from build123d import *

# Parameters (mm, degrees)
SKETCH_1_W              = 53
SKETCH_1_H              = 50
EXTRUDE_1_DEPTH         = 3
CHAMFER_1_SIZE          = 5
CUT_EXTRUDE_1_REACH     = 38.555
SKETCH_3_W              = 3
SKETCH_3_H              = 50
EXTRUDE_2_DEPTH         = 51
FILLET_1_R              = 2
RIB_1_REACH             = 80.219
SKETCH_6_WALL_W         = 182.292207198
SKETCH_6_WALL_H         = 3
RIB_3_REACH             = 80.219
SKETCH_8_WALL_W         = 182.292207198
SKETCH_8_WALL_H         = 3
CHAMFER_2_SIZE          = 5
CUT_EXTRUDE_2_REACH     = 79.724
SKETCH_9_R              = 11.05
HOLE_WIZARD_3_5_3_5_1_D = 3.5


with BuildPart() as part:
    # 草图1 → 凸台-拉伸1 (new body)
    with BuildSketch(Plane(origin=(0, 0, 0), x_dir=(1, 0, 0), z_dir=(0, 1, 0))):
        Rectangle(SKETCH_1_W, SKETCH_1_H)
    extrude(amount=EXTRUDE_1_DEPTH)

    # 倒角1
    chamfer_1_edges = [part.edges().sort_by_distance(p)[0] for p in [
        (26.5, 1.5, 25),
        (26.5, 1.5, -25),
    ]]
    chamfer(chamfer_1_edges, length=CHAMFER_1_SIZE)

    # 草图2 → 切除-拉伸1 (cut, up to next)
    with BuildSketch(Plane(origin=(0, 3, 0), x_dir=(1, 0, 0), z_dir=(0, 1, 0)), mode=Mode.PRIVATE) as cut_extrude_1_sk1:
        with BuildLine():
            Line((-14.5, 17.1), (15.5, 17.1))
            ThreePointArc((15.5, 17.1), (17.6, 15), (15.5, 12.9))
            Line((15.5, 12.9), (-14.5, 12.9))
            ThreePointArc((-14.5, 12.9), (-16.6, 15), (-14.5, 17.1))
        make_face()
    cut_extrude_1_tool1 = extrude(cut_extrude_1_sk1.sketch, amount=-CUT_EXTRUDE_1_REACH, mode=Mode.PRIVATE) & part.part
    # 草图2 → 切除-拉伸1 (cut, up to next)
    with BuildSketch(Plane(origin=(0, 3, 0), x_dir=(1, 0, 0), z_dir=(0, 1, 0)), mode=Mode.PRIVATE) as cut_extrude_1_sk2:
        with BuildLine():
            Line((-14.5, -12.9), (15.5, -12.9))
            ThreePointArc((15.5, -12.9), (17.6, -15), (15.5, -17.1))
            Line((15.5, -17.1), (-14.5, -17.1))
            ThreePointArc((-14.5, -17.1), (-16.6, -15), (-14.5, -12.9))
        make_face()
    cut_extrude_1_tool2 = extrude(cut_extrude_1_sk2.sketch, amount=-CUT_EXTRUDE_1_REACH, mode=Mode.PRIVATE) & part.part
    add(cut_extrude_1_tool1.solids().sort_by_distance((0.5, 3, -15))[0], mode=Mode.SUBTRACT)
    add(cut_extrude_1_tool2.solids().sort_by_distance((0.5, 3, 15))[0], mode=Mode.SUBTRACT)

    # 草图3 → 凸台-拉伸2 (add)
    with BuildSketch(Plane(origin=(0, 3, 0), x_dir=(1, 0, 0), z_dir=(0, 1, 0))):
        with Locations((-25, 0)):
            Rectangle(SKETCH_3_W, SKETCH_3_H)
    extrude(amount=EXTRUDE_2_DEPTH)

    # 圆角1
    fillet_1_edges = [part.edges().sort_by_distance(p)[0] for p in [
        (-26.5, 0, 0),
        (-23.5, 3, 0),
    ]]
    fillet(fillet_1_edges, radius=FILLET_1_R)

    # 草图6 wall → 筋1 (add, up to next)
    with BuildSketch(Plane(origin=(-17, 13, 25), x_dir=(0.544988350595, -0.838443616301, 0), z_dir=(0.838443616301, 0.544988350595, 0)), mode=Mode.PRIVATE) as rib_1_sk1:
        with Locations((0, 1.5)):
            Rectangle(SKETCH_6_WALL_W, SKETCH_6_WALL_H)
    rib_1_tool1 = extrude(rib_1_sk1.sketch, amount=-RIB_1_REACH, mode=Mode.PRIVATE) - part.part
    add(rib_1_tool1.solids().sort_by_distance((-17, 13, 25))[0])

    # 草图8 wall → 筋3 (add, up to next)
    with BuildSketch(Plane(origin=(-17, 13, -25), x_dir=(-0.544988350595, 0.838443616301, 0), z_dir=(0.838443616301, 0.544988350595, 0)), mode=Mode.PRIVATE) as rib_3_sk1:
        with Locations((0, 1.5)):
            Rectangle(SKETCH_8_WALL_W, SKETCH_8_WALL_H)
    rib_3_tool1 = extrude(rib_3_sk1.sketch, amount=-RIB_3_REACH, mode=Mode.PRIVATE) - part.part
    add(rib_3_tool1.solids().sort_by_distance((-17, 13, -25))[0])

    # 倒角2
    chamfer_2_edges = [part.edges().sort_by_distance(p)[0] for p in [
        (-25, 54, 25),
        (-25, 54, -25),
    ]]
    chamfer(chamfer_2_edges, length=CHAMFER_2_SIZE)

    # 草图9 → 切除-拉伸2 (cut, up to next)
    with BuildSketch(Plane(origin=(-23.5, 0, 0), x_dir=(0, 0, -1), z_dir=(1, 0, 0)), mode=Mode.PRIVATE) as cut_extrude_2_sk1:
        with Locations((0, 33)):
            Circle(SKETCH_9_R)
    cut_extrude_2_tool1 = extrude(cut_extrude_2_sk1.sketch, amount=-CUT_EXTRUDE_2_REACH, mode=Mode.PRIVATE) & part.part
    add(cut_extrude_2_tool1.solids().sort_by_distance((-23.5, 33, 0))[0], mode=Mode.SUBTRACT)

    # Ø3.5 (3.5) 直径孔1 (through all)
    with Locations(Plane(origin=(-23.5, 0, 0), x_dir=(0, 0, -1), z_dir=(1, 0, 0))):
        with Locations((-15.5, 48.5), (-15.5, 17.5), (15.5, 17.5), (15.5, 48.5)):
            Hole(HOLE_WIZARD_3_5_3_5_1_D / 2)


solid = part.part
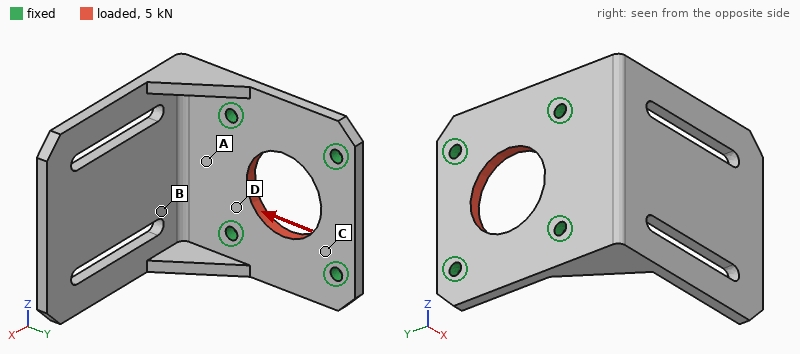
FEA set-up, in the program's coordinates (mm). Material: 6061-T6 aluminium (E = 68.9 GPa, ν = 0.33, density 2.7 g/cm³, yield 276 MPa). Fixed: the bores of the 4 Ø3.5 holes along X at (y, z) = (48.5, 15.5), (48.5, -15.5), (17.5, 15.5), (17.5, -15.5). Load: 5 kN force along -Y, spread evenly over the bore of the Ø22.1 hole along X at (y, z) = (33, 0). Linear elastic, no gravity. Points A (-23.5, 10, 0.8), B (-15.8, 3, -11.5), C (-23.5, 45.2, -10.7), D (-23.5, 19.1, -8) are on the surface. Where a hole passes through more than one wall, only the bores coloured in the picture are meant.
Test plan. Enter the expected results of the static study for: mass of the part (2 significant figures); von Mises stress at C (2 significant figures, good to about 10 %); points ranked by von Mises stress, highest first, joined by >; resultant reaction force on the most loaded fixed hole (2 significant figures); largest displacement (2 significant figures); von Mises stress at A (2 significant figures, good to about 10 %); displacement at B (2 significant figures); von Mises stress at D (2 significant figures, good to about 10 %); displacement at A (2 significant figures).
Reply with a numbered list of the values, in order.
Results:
1. 38 g
2. 36 MPa
3. C > D > A > B
4. 1.3 kN
5. 15 µm
6. 11 MPa
7. 3.7 µm
8. 21 MPa
9. 5.6 µm
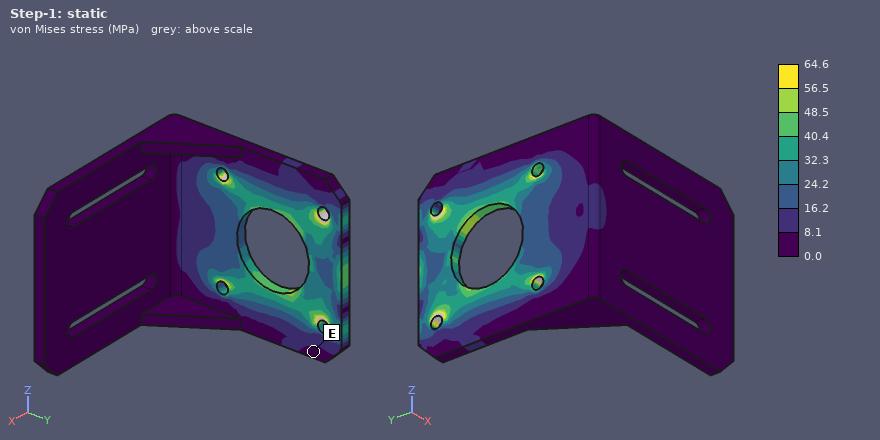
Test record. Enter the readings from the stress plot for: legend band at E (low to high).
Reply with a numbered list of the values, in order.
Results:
1. 0.0 to 8.1 MPa
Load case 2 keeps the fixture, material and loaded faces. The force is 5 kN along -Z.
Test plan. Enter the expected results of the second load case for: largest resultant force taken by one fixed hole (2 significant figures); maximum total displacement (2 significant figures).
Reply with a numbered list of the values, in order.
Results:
1. 1.3 kN
2. 12 µm
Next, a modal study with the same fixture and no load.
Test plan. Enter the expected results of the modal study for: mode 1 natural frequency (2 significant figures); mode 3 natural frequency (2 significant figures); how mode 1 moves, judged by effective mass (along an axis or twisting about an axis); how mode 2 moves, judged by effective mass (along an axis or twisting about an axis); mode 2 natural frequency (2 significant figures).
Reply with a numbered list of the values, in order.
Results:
1. 910 Hz
2. 3100 Hz
3. along Y
4. along Z
5. 1900 Hz
